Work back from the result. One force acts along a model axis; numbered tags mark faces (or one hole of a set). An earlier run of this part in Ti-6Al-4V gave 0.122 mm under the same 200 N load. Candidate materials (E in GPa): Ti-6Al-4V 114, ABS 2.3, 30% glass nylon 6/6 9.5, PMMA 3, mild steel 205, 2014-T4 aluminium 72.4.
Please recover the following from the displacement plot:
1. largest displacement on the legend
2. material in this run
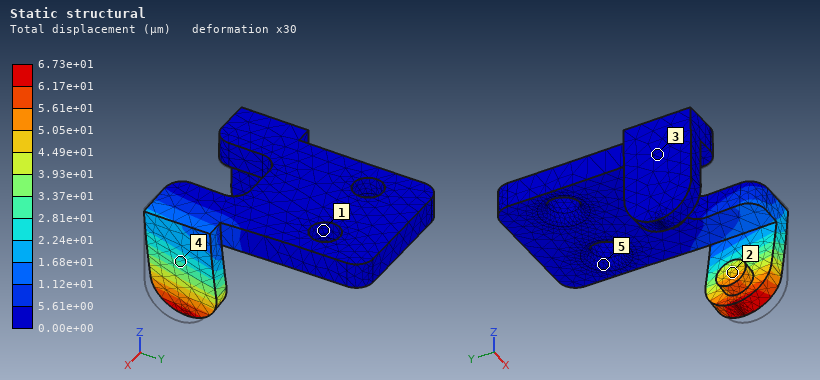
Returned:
6.73e+01 µm
mild steel
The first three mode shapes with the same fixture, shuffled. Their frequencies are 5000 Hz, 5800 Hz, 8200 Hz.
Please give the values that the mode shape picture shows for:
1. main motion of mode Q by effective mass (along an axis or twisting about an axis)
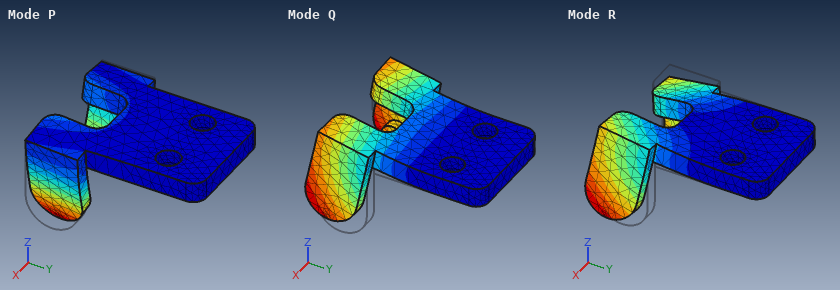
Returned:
along Z
